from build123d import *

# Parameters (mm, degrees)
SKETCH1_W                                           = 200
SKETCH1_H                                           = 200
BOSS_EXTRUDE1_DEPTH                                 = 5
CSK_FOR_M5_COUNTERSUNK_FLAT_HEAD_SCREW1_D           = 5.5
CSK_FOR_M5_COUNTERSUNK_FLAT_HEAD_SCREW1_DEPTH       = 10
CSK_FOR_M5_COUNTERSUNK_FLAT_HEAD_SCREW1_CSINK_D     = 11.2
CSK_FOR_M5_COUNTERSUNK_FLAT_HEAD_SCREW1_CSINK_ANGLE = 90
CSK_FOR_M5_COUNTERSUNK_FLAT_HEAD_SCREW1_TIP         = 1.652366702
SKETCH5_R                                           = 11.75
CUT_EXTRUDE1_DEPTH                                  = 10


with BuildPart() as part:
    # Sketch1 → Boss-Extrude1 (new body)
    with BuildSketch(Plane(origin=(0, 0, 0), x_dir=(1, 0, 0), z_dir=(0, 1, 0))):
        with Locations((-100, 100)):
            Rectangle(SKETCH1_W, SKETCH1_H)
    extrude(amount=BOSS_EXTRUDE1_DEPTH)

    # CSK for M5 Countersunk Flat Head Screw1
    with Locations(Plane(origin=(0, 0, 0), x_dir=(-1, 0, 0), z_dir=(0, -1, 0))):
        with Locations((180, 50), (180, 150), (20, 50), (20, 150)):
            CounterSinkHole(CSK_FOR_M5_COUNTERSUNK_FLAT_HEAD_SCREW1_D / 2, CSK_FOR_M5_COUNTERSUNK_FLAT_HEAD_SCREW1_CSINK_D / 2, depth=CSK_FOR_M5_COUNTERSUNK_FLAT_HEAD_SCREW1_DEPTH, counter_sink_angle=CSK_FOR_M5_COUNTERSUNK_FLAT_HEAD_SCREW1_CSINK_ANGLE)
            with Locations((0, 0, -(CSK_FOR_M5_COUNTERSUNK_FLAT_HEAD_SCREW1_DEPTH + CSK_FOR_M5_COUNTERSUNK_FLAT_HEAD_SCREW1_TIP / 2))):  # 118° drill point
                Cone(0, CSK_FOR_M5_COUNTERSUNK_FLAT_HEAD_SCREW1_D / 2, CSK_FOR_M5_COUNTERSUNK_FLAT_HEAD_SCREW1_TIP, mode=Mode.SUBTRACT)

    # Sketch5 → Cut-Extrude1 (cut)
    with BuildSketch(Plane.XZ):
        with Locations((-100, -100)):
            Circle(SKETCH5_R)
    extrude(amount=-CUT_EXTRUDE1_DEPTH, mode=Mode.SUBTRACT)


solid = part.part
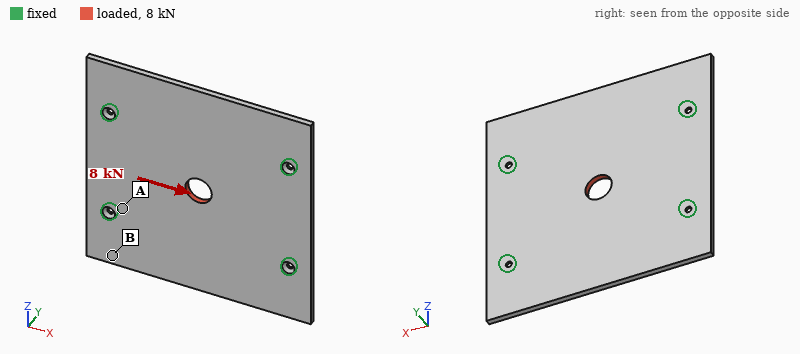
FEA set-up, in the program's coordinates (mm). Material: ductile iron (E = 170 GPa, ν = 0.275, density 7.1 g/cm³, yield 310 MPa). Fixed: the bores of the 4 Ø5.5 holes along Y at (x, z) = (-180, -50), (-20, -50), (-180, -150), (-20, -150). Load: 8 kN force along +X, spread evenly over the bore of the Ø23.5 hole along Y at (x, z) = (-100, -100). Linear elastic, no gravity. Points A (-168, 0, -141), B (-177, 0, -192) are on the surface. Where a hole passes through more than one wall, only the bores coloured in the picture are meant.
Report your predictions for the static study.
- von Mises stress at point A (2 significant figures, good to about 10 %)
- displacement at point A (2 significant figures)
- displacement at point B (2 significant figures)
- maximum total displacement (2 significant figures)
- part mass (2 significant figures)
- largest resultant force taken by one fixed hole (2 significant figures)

11 MPa
3.7 µm
2.9 µm
8.0 µm
1.4 kg
2.1 kN
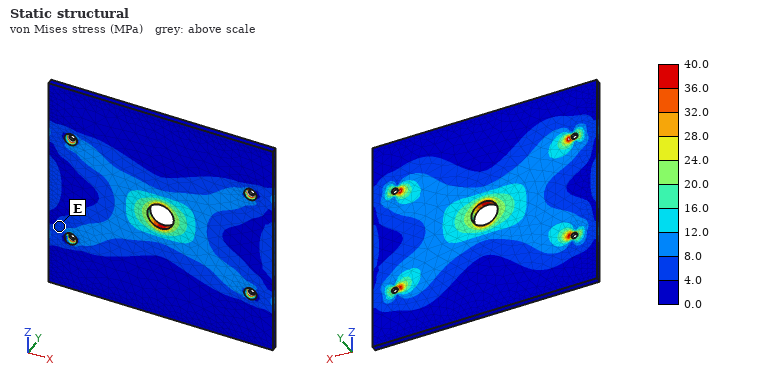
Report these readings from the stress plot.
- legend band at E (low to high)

4.0 to 8.0 MPa
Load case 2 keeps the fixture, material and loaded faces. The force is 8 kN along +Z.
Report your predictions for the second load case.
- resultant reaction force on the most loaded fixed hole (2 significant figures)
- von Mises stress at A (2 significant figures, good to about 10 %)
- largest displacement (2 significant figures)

2.1 kN
11 MPa
11 µm
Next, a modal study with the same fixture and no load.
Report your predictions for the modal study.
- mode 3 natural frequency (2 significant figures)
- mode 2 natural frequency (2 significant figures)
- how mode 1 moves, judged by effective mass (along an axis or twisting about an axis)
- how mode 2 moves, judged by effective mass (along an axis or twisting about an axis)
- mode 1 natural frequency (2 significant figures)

910 Hz
690 Hz
along Y
twisting about X
630 Hz
